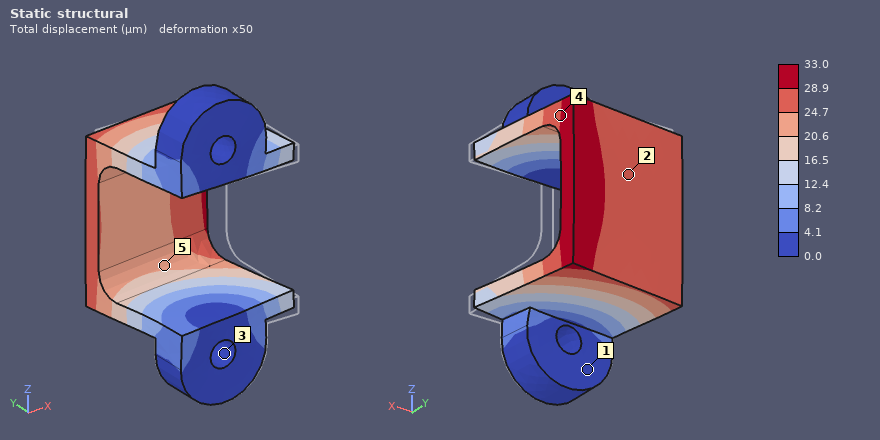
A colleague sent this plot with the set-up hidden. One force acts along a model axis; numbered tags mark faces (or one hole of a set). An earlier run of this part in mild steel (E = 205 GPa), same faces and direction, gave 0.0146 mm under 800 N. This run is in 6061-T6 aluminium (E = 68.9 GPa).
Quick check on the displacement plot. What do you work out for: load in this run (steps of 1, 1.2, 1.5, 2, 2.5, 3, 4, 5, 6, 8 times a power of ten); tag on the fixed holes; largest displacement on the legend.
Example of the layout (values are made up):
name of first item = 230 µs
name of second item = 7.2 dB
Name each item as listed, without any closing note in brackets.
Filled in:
load in this run = 600 N
tag on the fixed holes = 3
largest displacement on the legend = 33.0 µm
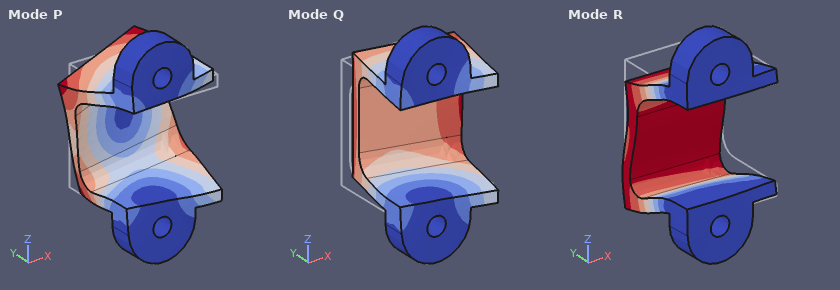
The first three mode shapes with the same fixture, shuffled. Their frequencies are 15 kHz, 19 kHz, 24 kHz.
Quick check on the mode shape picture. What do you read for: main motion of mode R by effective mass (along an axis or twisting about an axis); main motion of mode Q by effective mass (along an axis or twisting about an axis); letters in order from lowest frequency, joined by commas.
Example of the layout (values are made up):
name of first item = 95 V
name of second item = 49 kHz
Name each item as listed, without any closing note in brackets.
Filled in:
main motion of mode R by effective mass = along Z
main motion of mode Q by effective mass = along X
letters in order from lowest frequency, joined by commas = R, Q, P
